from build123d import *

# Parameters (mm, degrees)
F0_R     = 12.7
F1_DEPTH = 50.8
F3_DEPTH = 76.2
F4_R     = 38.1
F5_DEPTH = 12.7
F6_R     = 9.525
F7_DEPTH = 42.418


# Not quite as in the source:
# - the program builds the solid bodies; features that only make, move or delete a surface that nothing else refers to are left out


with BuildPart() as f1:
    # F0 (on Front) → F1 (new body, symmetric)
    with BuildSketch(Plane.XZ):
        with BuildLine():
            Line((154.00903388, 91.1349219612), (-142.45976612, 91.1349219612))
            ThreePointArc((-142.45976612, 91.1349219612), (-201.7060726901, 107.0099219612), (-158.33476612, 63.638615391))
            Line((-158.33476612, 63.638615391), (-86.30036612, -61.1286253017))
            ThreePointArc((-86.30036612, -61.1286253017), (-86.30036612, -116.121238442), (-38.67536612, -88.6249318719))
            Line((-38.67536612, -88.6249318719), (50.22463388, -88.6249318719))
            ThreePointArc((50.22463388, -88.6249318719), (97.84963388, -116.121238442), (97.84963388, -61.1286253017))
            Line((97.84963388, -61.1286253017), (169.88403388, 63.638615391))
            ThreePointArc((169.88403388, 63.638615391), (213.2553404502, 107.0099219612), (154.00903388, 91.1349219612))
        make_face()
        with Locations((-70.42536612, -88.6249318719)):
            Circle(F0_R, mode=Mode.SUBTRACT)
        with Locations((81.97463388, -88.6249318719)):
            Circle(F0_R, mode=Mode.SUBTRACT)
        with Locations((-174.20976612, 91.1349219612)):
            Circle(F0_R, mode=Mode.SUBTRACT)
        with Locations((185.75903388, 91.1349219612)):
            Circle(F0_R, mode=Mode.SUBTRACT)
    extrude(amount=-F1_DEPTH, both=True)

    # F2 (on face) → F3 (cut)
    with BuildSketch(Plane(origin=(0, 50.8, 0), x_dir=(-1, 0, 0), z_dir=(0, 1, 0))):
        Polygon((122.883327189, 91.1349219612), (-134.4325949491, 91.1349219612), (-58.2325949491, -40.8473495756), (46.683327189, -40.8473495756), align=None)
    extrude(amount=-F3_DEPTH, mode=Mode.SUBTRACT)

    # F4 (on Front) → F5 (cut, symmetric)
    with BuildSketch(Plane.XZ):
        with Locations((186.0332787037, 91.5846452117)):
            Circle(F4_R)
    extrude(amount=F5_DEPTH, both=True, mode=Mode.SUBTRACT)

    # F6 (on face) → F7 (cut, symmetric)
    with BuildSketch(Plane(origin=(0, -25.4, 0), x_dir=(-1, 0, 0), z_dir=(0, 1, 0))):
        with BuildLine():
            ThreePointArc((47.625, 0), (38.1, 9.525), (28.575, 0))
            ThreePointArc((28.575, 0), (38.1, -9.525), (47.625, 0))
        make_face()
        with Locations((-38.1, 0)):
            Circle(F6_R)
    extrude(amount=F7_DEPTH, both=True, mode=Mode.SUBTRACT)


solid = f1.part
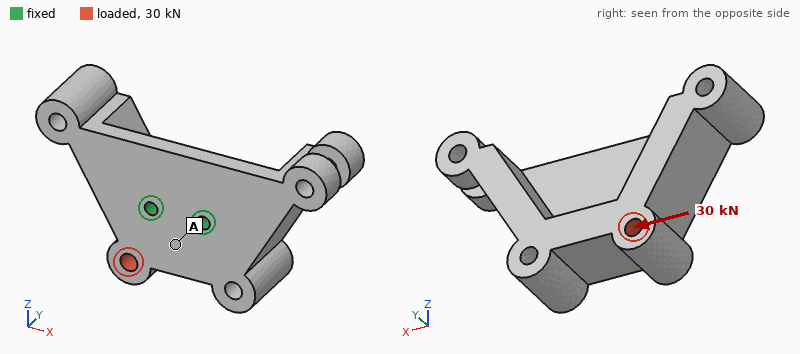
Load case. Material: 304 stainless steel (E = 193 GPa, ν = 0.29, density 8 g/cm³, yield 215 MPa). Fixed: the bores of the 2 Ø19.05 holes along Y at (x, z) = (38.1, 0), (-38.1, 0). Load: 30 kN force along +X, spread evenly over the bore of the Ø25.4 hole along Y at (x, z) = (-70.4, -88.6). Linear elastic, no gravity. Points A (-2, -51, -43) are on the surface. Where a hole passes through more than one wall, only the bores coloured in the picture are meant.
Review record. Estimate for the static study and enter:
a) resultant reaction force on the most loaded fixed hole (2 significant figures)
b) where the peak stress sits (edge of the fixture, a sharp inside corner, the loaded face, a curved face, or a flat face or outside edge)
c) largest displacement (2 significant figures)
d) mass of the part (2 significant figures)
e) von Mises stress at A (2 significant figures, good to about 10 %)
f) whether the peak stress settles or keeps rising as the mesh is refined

35 kN
edge of the fixture
39 µm
28 kg
11 MPa
keeps rising
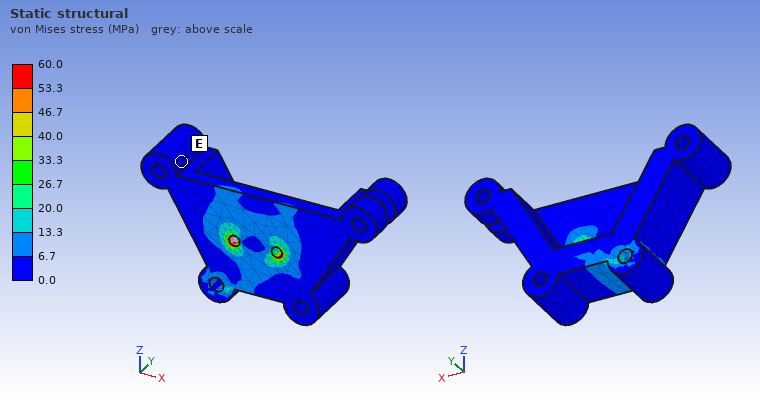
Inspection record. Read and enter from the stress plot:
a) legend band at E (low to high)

0.0 to 6.7 MPa
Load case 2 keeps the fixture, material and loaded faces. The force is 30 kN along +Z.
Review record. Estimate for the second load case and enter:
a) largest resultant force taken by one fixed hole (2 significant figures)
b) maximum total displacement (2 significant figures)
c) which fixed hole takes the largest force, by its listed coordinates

39 kN
88 µm
(-38.1, 0)
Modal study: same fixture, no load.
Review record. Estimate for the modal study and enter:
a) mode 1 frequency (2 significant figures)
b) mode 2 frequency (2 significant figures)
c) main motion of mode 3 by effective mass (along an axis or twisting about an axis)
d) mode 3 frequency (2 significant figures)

590 Hz
740 Hz
twisting about Y
1100 Hz
